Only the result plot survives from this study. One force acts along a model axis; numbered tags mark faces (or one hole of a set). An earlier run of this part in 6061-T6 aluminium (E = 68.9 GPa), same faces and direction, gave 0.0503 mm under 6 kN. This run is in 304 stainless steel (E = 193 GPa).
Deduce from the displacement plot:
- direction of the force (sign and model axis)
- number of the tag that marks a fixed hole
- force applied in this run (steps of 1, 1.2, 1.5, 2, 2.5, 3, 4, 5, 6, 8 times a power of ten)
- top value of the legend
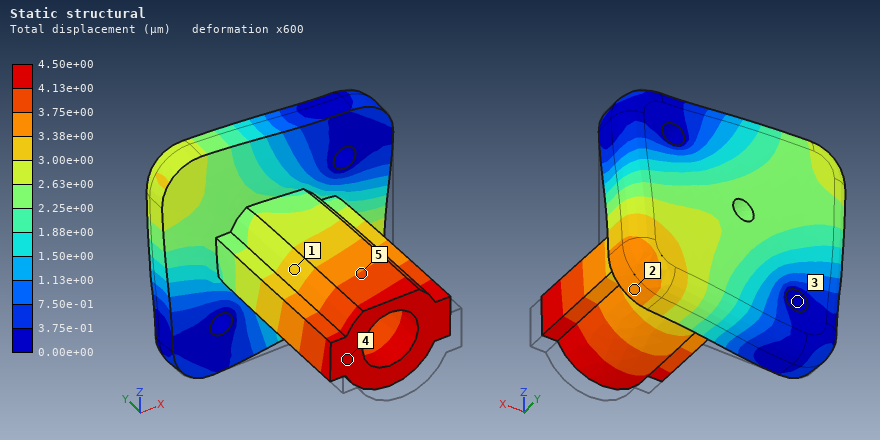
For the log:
+Y
3
1.5 kN
4.50e+00 µm
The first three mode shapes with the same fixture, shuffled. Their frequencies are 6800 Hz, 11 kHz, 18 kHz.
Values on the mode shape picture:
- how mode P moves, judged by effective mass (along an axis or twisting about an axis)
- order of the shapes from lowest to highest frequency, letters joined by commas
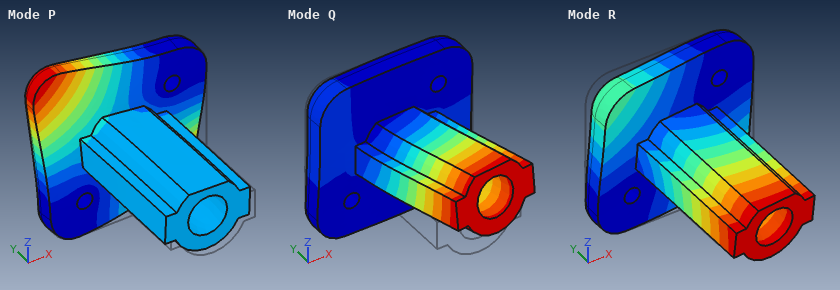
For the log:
along Y
R, Q, P
